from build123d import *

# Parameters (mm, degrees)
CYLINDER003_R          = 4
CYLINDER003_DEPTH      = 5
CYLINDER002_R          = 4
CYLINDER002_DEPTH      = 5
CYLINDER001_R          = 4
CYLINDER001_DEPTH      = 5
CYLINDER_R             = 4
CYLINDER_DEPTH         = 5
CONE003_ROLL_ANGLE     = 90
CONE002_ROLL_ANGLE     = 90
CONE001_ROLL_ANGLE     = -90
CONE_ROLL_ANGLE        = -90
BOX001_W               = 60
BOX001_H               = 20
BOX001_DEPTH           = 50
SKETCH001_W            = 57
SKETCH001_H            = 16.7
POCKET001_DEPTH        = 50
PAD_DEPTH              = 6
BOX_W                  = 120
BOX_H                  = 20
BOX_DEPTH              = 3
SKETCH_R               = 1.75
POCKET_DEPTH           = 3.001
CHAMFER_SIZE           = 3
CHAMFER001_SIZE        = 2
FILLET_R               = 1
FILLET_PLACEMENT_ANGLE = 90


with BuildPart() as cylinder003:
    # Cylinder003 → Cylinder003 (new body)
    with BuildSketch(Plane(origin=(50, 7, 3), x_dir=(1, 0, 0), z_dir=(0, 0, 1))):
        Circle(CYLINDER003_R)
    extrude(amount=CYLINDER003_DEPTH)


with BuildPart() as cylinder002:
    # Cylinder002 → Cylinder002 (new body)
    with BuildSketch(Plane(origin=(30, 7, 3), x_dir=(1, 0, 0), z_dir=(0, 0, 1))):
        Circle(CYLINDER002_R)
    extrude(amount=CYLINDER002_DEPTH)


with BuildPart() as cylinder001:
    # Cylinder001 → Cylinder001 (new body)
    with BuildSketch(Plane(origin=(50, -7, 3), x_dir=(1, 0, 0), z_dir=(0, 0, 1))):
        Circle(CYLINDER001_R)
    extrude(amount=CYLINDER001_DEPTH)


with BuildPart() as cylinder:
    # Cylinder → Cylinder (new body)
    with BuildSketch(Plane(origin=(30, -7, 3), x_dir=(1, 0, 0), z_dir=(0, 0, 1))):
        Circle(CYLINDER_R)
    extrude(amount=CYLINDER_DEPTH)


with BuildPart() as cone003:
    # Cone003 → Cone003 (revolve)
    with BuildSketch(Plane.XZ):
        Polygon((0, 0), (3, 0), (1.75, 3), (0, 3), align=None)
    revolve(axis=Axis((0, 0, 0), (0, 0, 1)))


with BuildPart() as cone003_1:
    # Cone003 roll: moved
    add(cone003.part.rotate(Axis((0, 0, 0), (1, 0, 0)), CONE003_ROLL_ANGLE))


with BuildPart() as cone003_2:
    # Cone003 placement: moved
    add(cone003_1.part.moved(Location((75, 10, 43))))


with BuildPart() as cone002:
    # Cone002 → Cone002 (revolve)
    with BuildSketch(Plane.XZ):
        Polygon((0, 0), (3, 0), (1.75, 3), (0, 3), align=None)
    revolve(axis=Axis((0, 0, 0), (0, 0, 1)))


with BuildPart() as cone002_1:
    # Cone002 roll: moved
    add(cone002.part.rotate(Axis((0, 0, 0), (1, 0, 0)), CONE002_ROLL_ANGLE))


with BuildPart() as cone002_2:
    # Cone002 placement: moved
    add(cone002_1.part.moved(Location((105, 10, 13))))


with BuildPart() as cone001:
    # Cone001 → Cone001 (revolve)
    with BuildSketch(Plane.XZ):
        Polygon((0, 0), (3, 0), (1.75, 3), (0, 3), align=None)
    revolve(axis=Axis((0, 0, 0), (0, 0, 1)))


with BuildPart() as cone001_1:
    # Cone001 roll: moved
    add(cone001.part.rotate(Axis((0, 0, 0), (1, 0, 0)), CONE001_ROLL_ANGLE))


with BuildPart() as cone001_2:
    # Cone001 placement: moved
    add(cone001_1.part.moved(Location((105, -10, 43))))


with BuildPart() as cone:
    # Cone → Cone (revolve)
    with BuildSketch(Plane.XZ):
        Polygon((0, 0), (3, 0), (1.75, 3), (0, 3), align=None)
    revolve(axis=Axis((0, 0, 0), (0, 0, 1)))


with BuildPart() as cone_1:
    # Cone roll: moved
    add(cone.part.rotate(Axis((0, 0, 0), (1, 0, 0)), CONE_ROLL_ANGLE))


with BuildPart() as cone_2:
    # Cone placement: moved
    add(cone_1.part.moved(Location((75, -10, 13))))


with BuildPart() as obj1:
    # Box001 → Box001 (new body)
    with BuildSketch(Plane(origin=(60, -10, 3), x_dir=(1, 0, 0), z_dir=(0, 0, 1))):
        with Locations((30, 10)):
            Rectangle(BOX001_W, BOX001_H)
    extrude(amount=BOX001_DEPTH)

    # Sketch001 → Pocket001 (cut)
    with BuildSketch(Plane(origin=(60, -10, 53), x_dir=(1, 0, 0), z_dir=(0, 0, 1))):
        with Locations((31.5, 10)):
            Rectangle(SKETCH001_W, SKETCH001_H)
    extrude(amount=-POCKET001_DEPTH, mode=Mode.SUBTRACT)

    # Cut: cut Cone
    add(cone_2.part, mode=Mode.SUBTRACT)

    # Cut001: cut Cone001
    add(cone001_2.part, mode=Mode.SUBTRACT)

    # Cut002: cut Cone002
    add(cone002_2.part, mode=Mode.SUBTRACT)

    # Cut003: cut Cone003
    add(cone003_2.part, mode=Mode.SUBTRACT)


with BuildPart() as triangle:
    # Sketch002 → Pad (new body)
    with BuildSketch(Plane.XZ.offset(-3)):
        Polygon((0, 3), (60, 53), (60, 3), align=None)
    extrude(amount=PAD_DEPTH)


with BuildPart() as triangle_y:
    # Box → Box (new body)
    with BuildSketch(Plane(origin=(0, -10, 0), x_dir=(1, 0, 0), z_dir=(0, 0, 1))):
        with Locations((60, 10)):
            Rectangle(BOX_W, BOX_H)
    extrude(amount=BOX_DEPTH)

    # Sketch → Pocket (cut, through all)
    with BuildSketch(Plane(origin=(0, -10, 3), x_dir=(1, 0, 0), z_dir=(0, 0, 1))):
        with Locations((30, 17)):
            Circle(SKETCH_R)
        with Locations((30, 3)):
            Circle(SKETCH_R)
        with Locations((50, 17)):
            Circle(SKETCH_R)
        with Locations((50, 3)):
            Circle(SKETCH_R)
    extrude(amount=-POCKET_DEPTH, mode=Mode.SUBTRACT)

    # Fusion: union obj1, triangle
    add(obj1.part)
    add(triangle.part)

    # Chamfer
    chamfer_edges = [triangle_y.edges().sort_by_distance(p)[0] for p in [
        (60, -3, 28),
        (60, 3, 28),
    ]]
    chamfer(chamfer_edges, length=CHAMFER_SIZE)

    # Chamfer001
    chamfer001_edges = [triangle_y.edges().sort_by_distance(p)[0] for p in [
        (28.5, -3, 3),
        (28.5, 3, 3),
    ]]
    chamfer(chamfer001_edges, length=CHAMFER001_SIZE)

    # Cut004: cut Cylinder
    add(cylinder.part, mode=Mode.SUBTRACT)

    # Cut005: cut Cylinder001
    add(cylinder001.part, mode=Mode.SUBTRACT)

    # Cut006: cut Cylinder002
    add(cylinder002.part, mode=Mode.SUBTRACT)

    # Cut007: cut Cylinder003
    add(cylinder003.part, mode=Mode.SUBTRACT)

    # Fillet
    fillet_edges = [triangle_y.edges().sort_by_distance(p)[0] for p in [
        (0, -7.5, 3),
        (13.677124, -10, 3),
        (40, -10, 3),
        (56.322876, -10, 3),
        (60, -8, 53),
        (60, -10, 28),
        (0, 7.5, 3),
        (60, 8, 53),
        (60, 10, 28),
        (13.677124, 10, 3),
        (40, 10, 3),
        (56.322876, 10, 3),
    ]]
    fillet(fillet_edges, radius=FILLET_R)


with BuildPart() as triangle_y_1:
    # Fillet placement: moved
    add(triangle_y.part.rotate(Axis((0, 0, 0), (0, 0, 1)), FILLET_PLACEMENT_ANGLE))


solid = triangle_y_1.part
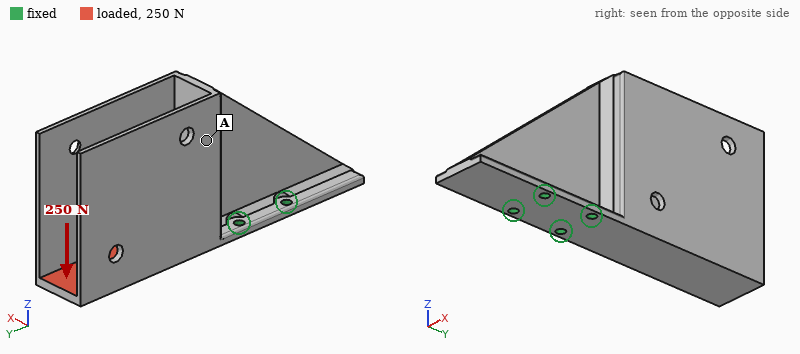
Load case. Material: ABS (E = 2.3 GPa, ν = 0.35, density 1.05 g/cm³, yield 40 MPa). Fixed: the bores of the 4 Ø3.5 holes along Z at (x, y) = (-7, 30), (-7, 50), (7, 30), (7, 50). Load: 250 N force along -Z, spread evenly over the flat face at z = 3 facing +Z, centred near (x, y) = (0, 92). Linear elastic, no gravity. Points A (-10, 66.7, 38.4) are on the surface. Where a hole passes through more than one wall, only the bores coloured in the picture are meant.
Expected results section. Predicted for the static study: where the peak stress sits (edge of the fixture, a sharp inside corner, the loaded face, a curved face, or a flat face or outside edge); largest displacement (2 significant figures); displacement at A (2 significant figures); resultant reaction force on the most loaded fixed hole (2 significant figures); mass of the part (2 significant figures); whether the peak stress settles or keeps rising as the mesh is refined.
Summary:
edge of the fixture
1.4 mm
0.57 mm
380 N
30 g
keeps rising
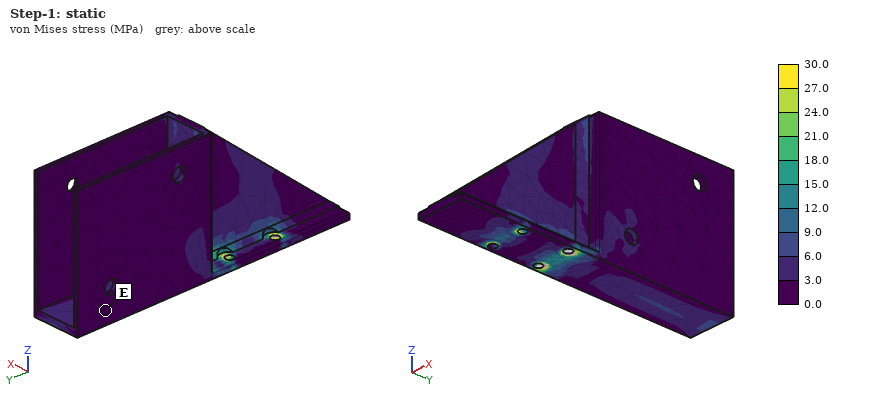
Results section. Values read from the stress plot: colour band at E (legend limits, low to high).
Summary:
0.0 to 3.0 MPa
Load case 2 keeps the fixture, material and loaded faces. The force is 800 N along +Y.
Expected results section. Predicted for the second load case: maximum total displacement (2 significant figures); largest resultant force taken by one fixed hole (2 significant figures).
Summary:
0.20 mm
330 N
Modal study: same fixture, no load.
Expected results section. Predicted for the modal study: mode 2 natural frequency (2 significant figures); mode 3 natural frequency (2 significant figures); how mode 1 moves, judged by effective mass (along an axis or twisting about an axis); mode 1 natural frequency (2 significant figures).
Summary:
270 Hz
610 Hz
along X
250 Hz
